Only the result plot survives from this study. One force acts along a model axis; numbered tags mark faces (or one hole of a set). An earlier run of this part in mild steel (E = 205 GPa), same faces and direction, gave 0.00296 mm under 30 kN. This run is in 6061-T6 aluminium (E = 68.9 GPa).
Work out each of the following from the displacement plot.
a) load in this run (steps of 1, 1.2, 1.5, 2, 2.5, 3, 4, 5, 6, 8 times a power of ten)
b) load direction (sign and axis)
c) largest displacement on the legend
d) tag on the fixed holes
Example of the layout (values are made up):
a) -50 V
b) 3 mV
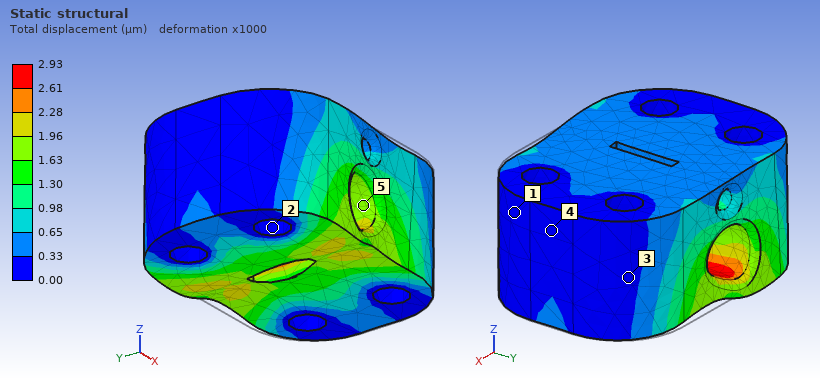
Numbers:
a) 10 kN
b) -X
c) 2.93 µm
d) 2
